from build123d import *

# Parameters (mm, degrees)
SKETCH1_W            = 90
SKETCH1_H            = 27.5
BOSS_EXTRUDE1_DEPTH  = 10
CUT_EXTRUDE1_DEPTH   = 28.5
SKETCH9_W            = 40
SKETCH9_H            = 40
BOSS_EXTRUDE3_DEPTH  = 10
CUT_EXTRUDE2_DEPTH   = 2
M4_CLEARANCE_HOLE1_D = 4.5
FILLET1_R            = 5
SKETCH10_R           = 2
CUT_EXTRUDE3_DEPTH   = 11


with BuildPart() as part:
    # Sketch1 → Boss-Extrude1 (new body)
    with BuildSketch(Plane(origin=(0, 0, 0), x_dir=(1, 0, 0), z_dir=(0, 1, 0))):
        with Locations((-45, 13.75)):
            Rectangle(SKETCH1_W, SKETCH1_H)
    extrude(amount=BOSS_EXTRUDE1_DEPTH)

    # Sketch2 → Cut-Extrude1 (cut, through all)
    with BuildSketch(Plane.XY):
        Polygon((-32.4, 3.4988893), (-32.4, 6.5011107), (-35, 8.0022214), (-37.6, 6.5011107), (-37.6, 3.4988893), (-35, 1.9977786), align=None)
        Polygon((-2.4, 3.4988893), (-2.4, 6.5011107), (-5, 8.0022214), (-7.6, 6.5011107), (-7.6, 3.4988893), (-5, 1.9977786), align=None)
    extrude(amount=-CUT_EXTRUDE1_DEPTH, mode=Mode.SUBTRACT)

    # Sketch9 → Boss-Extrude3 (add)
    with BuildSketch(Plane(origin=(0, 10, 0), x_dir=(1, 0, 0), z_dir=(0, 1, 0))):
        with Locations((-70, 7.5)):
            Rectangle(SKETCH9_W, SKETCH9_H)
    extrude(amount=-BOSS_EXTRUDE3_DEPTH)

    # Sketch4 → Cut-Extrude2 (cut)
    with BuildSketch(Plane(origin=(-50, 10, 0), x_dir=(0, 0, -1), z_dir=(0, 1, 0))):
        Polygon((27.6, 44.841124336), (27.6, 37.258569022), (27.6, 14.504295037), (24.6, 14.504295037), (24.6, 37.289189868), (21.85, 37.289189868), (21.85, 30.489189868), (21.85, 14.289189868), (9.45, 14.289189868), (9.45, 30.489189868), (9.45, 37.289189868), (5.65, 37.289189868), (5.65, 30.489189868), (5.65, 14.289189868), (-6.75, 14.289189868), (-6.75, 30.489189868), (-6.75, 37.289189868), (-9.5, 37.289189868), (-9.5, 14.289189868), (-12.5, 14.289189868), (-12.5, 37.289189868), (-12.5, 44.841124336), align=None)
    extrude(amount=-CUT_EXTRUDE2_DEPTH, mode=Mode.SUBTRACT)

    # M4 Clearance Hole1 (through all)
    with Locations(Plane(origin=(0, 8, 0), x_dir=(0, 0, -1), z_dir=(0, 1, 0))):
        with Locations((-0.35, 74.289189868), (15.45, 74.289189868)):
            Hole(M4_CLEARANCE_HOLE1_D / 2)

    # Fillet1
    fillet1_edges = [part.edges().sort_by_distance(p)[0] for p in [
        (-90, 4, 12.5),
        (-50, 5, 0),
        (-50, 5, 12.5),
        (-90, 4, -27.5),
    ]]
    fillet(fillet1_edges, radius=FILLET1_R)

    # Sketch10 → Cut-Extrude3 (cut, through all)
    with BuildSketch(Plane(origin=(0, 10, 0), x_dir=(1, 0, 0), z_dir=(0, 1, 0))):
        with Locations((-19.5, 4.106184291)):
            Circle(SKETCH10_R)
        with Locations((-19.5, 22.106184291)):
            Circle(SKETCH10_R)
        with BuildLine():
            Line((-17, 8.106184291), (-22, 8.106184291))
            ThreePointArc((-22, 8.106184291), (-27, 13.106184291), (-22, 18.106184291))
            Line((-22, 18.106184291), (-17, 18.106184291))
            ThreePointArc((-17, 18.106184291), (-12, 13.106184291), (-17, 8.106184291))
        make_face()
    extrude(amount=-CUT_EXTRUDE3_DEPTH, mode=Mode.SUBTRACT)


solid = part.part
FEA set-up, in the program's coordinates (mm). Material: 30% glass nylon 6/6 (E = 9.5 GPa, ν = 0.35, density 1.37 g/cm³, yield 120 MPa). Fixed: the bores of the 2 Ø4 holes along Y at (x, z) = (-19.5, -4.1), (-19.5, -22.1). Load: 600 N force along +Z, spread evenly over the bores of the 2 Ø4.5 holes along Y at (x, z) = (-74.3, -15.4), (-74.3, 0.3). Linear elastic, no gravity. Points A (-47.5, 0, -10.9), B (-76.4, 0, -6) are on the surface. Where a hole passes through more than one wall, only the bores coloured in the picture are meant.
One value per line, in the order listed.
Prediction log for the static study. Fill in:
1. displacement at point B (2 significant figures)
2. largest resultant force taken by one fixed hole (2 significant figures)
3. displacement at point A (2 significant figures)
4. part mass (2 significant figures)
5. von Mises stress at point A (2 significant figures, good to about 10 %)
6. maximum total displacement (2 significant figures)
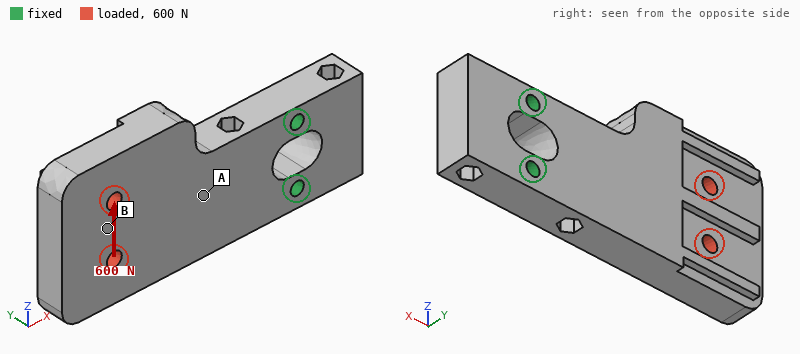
0.32 mm
1.6 kN
0.11 mm
34 g
8.2 MPa
0.43 mm
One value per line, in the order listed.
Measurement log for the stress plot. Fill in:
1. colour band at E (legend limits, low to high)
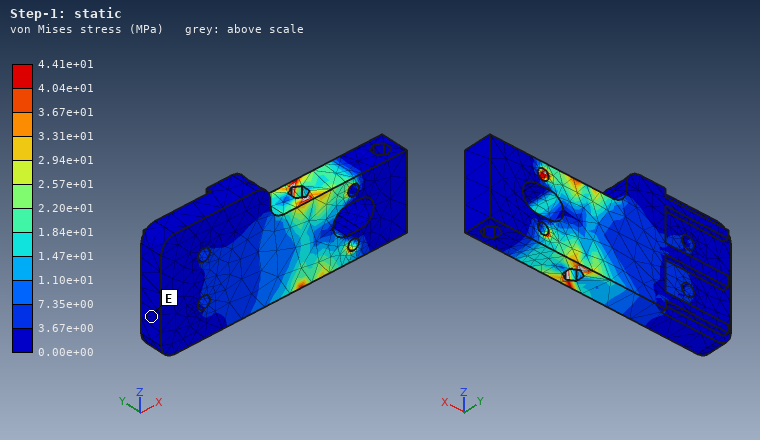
0.00e+00 to 3.67e+00 MPa
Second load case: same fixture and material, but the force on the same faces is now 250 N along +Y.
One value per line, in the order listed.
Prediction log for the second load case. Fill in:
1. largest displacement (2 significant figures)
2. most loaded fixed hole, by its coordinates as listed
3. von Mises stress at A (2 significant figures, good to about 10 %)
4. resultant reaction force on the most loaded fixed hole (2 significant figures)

1.1 mm
(-19.5, -4.1)
14 MPa
180 N
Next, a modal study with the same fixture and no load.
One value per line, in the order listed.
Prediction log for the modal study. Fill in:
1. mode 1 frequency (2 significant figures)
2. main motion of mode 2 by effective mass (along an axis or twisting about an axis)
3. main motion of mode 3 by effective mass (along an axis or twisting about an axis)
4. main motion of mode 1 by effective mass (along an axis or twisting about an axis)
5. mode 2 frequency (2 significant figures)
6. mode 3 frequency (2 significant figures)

700 Hz
along Z
twisting about X
along Y
1700 Hz
2300 Hz
